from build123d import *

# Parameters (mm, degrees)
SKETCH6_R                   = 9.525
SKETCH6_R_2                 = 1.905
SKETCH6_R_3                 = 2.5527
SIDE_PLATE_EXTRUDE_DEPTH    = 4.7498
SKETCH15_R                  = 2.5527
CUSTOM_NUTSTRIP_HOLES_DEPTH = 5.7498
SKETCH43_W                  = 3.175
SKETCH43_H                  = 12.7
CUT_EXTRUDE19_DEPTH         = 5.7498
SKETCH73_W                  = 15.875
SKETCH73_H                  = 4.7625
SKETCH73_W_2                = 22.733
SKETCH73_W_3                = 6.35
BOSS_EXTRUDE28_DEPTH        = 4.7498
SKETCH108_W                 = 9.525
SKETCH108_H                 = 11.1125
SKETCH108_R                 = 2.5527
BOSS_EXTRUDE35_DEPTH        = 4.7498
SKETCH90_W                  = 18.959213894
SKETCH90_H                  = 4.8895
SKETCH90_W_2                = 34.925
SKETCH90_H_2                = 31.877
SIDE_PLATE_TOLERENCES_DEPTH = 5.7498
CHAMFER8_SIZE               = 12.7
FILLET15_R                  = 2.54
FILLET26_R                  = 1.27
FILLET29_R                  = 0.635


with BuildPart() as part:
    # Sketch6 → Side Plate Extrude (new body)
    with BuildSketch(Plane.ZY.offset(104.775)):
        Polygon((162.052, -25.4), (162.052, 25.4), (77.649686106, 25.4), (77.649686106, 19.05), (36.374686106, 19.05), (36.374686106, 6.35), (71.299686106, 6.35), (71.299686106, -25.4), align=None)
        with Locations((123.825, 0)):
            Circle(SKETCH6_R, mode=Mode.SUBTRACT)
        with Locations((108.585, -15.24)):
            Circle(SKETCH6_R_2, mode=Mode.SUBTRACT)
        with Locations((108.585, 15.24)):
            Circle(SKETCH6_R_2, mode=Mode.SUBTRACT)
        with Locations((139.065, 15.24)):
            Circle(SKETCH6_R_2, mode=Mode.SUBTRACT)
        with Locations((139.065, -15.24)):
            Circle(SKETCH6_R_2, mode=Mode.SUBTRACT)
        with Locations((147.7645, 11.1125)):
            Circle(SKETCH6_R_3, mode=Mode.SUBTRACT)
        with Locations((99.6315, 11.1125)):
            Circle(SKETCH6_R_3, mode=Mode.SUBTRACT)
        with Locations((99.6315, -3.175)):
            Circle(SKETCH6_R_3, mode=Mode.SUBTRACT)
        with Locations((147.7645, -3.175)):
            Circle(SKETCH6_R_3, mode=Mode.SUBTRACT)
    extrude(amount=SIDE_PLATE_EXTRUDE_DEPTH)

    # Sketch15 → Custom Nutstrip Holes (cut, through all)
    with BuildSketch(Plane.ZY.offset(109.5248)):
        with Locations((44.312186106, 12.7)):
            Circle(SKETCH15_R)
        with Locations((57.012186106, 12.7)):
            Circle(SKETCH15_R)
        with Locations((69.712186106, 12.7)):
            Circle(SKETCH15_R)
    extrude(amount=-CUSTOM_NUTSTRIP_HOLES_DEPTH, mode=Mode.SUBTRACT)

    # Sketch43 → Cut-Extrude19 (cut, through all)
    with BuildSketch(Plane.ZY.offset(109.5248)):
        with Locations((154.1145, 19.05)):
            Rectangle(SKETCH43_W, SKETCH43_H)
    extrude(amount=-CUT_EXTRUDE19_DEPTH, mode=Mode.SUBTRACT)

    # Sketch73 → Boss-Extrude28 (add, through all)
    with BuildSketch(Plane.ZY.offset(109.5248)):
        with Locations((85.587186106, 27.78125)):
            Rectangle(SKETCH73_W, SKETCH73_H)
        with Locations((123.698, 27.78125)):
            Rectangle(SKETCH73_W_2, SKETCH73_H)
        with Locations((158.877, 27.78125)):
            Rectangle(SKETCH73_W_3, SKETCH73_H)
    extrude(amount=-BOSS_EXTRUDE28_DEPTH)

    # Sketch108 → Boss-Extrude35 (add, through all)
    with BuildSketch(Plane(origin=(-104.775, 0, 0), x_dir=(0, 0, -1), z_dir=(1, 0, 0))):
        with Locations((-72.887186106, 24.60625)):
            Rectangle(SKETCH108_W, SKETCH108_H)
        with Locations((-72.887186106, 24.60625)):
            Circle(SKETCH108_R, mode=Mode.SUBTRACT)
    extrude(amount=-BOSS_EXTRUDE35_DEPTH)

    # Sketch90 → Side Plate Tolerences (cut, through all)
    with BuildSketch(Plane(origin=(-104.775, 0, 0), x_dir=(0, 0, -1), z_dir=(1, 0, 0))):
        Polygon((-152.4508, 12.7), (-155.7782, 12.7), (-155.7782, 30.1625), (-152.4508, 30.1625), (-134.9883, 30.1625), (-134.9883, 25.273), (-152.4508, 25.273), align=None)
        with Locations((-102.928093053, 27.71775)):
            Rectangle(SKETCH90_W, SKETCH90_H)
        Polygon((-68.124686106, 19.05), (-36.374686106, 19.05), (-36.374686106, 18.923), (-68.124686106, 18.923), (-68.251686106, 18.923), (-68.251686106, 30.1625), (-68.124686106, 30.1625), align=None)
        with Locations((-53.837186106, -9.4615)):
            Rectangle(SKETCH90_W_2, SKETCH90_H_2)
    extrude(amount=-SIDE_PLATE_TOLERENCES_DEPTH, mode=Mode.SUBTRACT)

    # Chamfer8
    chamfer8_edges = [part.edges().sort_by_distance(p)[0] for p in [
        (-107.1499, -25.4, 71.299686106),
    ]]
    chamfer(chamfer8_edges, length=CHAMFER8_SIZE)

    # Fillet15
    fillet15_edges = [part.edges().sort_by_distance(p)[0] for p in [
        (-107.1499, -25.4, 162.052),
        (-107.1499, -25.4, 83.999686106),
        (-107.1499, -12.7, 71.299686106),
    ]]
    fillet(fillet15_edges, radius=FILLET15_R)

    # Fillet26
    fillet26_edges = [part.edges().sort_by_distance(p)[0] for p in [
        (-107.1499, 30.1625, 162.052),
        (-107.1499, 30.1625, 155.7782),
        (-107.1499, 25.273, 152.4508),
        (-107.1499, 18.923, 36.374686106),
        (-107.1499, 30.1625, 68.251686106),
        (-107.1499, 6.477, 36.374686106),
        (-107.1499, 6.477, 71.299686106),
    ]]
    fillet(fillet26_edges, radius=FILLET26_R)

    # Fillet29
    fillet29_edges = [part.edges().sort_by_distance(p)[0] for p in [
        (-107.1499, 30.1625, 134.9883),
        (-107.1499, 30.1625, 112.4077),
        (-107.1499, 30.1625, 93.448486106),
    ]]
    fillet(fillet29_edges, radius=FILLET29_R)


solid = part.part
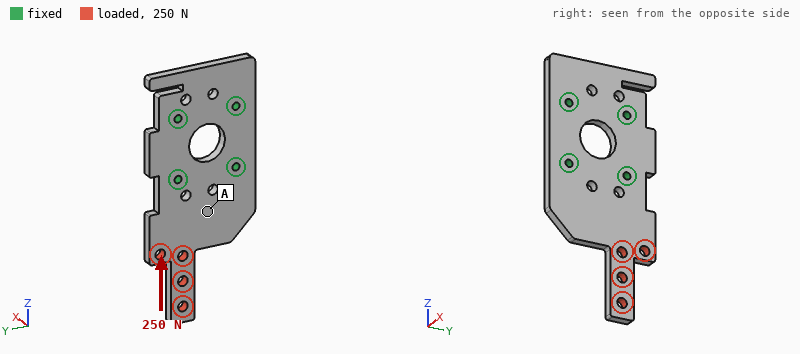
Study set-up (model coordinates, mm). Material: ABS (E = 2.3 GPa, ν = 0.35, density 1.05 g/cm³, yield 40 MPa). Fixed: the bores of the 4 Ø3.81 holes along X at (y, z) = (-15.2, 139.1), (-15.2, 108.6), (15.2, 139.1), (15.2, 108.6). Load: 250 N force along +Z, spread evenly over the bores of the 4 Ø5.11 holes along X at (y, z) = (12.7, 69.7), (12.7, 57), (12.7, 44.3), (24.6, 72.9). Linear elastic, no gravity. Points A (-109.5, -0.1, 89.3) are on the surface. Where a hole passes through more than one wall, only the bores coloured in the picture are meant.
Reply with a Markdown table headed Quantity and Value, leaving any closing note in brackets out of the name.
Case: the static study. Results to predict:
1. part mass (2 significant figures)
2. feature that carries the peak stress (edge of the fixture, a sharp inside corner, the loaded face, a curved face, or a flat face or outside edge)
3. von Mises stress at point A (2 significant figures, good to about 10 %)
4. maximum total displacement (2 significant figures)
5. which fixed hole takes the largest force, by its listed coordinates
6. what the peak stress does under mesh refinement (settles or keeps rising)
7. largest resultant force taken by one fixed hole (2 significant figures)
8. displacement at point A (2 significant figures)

| Quantity | Value |
|---|---|
| part mass | 23 g |
| feature that carries the peak stress | edge of the fixture |
| von Mises stress at point A | 0.75 MPa |
| maximum total displacement | 0.10 mm |
| which fixed hole takes the largest force, by its listed coordinates | (15.2, 108.6) |
| what the peak stress does under mesh refinement | keeps rising |
| largest resultant force taken by one fixed hole | 200 N |
| displacement at point A | 0.016 mm |
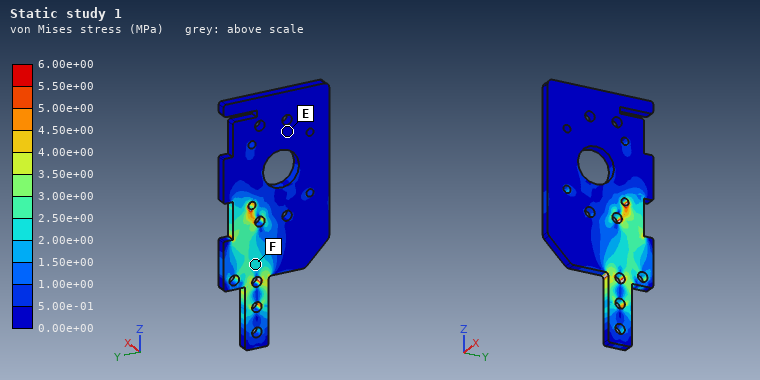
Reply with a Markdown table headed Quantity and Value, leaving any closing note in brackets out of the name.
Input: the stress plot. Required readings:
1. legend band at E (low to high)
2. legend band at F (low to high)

| Quantity | Value |
|---|---|
| legend band at E | 0.00e+00 to 5.00e-01 MPa |
| legend band at F | 2.00e+00 to 2.50e+00 MPa |
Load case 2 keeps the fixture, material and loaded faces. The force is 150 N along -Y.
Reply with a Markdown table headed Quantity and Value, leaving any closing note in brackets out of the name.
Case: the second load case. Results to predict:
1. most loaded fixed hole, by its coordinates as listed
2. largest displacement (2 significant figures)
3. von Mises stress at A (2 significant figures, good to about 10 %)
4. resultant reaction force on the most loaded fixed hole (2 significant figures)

| Quantity | Value |
|---|---|
| most loaded fixed hole, by its coordinates as listed | (-15.2, 108.6) |
| largest displacement | 0.62 mm |
| von Mises stress at A | 2.4 MPa |
| resultant reaction force on the most loaded fixed hole | 200 N |
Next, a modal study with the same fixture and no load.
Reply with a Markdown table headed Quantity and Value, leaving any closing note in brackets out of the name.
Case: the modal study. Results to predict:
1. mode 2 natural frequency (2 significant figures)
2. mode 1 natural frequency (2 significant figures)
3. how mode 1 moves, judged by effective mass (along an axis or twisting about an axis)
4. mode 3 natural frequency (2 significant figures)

| Quantity | Value |
|---|---|
| mode 2 natural frequency | 1100 Hz |
| mode 1 natural frequency | 350 Hz |
| how mode 1 moves, judged by effective mass | along X |
| mode 3 natural frequency | 1400 Hz |
